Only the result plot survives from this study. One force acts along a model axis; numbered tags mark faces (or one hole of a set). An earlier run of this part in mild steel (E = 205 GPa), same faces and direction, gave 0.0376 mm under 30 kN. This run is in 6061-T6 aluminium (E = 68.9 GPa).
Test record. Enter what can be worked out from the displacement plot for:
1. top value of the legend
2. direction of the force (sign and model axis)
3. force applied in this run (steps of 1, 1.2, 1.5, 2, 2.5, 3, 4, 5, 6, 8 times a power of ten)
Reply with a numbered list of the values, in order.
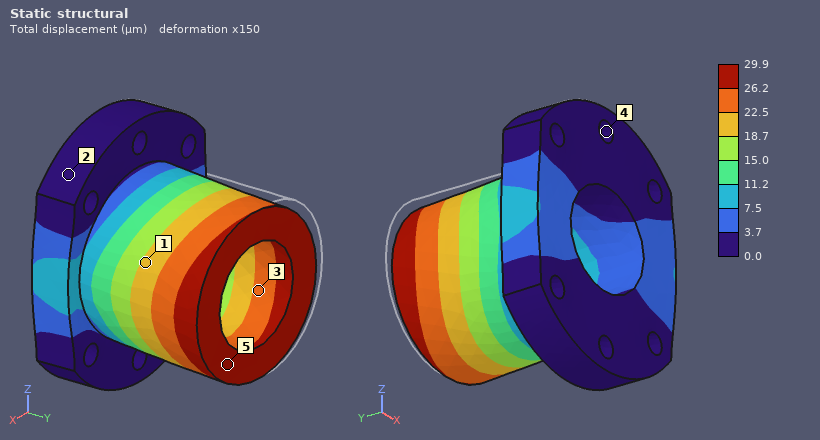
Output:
1. 29.9 µm
2. +X
3. 8 kN
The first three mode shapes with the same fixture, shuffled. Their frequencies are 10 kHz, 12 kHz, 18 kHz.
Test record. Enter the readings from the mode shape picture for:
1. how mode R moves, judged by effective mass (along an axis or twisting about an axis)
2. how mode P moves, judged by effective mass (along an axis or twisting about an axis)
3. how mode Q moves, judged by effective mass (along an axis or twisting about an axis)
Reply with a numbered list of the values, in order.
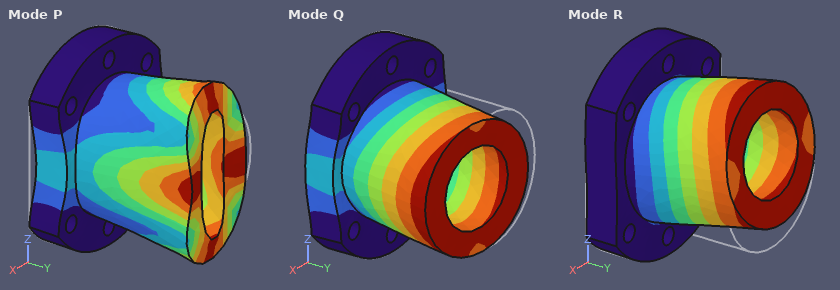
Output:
1. along Z
2. along Y
3. along X
